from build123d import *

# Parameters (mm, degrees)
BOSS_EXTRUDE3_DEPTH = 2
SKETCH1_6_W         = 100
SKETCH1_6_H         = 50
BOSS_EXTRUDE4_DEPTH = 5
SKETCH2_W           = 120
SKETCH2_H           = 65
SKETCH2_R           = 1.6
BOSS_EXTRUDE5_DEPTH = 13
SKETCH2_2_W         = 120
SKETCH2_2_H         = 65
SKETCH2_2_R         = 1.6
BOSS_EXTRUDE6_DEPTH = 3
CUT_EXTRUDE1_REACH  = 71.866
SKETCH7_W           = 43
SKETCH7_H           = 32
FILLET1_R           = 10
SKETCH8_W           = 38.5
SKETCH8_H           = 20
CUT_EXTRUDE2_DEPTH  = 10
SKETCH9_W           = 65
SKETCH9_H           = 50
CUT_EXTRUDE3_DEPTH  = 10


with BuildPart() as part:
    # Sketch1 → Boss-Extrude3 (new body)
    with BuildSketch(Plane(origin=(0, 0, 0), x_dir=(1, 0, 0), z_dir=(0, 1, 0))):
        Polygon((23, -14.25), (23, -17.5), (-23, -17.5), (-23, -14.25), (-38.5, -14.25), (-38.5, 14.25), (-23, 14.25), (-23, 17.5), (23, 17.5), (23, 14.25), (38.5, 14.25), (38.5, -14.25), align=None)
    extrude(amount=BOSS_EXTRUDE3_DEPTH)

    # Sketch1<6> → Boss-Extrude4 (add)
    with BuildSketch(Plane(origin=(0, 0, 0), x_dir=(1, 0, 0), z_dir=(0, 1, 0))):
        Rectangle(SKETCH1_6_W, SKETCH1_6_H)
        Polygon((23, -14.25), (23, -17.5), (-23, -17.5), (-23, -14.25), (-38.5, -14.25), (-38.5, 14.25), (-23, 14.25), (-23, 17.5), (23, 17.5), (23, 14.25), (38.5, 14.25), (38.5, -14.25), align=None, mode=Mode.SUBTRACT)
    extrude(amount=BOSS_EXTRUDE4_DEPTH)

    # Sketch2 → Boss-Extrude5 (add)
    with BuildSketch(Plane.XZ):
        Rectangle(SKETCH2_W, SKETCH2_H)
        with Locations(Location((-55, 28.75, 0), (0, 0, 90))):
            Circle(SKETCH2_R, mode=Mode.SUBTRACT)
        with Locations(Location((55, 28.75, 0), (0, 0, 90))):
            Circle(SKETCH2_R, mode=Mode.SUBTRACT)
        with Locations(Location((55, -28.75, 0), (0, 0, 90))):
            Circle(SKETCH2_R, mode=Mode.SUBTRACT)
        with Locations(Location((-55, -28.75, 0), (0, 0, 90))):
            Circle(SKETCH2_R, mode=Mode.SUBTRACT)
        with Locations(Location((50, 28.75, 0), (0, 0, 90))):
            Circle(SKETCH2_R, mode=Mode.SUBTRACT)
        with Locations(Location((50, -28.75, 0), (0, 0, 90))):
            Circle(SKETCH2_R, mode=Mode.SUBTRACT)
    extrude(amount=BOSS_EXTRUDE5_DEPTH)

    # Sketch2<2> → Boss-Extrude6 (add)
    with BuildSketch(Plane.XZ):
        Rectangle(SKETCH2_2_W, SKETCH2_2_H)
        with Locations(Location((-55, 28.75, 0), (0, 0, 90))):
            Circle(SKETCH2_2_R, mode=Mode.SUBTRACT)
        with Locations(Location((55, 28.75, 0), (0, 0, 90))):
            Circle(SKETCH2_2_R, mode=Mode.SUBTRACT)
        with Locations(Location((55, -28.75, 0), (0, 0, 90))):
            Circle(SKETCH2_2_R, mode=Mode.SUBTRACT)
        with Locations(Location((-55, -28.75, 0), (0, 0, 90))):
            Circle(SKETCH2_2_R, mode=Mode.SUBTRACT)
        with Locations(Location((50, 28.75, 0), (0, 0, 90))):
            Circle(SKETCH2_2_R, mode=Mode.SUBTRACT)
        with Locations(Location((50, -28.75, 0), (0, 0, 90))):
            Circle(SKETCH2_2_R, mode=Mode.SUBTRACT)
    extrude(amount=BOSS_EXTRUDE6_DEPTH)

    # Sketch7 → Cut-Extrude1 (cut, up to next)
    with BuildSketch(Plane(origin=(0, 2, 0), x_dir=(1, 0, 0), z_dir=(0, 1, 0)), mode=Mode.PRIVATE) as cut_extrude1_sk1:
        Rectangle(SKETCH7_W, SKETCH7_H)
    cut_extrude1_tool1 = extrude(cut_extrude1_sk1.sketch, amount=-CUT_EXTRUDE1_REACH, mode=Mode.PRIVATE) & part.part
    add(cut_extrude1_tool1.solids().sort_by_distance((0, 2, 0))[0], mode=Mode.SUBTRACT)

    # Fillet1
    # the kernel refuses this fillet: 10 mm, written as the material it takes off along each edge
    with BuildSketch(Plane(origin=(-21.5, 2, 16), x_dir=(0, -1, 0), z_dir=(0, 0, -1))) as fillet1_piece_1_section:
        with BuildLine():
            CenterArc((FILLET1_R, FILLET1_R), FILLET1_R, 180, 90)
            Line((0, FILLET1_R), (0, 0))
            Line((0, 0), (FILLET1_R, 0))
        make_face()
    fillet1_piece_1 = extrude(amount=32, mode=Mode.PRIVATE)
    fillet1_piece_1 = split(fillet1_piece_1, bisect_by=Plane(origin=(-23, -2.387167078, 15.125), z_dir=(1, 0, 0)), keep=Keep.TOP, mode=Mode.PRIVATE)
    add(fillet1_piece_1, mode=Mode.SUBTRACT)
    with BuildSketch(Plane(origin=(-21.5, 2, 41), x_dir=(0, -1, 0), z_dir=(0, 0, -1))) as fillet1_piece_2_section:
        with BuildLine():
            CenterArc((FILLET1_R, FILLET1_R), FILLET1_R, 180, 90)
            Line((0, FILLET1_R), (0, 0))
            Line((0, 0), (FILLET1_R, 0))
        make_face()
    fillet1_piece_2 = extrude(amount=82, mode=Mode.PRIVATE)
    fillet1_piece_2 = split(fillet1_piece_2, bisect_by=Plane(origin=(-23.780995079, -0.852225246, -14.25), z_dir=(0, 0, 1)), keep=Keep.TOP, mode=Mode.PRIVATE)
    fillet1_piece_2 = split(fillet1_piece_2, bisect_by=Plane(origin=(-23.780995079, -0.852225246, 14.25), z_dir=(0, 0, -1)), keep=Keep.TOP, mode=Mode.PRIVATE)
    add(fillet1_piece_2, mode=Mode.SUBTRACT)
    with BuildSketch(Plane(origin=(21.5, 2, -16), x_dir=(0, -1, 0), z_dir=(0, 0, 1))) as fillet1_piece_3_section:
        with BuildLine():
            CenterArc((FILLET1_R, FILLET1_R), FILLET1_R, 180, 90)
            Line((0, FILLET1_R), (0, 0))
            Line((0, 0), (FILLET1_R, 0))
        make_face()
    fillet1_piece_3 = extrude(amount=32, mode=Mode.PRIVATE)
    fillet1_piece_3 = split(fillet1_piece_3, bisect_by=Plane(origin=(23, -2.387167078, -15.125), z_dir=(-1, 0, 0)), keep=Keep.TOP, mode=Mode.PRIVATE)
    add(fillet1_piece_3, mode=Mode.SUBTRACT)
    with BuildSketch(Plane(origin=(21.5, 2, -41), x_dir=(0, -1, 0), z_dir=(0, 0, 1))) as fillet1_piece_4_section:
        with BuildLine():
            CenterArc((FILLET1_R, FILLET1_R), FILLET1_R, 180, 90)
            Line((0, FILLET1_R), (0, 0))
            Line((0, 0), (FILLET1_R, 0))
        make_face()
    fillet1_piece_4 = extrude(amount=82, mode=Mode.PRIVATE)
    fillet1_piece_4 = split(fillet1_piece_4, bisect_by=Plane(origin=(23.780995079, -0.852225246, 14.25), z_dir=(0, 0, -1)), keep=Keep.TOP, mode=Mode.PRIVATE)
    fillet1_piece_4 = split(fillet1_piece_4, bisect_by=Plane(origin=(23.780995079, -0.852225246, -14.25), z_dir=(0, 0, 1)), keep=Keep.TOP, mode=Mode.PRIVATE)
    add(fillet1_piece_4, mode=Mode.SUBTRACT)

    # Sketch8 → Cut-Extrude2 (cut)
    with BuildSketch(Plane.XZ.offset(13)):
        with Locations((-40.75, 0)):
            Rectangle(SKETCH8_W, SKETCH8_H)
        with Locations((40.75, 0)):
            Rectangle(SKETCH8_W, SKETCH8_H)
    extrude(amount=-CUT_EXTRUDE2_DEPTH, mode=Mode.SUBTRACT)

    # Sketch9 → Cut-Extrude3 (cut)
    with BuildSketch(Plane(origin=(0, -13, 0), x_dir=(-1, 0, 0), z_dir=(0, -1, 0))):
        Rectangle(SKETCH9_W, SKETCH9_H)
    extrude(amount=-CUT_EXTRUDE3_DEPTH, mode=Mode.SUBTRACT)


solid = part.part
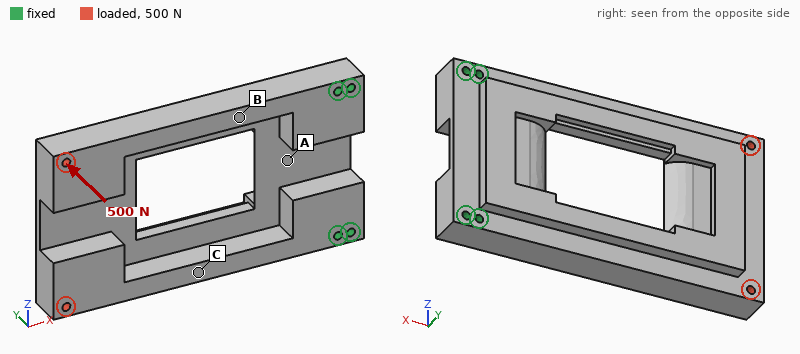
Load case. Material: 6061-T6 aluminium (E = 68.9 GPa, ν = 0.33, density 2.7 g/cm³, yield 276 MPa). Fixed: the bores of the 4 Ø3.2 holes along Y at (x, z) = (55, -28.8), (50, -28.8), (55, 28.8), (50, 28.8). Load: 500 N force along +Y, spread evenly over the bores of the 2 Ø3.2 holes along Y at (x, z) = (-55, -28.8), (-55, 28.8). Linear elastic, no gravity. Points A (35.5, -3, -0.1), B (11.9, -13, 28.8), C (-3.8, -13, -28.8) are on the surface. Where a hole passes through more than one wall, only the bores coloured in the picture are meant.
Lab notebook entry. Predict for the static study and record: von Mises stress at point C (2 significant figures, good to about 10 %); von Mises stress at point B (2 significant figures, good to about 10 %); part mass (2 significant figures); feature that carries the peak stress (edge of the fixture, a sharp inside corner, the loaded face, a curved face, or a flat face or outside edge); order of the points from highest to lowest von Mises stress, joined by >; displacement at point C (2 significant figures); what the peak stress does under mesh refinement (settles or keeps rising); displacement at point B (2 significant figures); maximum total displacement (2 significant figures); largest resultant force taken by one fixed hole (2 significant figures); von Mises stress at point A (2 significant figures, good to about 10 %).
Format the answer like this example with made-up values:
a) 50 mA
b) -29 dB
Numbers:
a) 32 MPa
b) 42 MPa
c) 180 g
d) edge of the fixture
e) B > C > A
f) 0.14 mm
g) keeps rising
h) 0.079 mm
i) 0.42 mm
j) 1.0 kN
k) 8.8 MPa
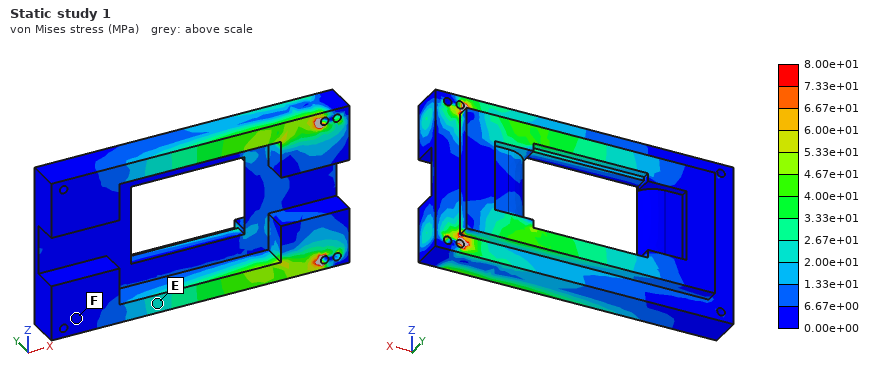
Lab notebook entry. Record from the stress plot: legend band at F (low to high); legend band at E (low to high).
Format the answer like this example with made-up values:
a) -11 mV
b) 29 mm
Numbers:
a) 0.00e+00 to 6.67e+00 MPa
b) 2.00e+01 to 2.67e+01 MPa
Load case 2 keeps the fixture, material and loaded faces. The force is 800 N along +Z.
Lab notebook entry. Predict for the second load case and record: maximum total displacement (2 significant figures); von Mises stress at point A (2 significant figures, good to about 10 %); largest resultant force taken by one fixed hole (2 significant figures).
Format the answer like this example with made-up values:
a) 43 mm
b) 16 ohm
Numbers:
a) 0.17 mm
b) 14 MPa
c) 1.3 kN
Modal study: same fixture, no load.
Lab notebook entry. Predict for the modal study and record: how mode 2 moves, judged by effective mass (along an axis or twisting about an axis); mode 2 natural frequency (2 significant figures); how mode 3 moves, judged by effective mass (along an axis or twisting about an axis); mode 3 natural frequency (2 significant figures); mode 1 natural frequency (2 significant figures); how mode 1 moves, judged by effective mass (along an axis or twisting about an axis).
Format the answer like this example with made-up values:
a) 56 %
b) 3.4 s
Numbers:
a) along Z
b) 1300 Hz
c) along Z
d) 2200 Hz
e) 760 Hz
f) along Y
